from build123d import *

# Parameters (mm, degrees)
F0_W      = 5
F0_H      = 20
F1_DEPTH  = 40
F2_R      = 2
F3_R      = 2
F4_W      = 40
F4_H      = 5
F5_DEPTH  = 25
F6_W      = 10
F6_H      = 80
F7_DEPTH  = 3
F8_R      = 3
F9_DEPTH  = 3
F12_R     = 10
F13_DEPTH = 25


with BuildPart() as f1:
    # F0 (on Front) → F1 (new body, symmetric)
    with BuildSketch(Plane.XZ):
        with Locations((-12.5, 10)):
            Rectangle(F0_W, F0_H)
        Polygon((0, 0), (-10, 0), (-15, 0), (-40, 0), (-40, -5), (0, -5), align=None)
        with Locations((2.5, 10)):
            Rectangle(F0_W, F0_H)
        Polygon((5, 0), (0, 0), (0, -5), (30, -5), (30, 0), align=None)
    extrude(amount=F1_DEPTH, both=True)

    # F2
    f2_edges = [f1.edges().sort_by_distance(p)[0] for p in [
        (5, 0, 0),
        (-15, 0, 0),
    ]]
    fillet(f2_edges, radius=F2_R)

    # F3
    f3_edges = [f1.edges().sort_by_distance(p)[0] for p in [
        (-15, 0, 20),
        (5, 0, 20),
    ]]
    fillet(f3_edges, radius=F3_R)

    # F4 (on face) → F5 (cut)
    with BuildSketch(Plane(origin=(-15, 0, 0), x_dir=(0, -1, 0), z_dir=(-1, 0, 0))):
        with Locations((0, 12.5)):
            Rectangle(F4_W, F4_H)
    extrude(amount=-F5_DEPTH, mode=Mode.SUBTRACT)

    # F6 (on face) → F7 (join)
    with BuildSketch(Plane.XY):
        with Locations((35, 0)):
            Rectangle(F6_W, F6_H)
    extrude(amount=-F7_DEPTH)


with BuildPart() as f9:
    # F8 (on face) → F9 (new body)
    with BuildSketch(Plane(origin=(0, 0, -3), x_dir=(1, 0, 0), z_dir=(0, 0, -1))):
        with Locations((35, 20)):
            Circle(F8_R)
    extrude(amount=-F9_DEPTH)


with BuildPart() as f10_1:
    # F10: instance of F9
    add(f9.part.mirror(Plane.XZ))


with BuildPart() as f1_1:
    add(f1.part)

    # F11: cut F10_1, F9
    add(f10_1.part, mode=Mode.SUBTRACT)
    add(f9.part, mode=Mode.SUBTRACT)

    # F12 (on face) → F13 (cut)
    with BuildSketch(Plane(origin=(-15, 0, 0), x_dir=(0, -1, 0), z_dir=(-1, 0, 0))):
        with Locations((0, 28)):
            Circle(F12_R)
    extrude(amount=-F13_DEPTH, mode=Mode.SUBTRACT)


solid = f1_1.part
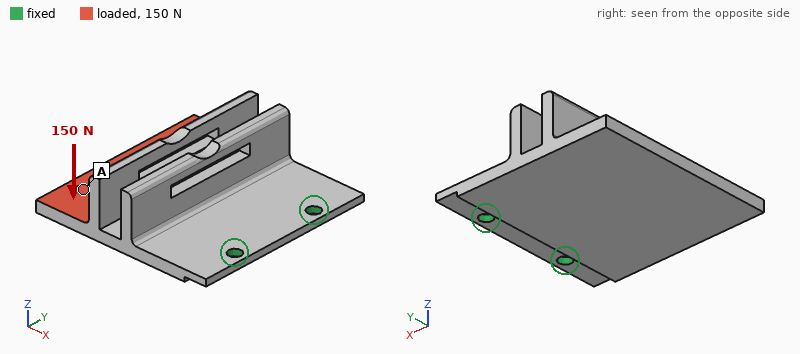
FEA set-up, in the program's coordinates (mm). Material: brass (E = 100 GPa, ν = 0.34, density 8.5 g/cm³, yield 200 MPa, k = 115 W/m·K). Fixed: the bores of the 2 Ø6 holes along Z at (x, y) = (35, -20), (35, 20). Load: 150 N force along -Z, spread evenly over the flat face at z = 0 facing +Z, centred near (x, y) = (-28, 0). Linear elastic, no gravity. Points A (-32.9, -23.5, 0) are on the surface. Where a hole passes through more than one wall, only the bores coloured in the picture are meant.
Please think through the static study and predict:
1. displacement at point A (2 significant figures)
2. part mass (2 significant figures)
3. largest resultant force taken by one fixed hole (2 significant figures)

0.34 mm
370 g
76 N
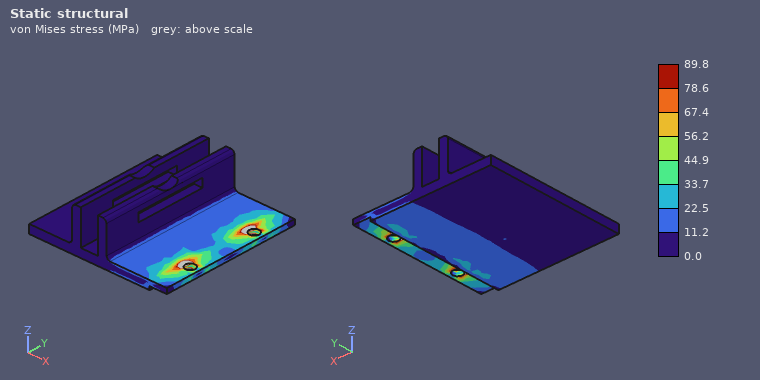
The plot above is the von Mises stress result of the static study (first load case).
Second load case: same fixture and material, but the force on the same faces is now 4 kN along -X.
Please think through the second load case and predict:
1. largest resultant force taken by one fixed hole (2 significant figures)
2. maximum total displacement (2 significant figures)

2.0 kN
0.40 mm
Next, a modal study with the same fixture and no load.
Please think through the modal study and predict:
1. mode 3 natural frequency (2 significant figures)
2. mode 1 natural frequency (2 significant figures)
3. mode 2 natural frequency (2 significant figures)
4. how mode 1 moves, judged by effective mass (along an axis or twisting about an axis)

2000 Hz
280 Hz
800 Hz
along Z
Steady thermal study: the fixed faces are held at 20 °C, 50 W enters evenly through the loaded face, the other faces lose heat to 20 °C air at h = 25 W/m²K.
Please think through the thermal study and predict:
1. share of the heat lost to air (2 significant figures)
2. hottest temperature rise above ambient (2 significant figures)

33 %
61 K
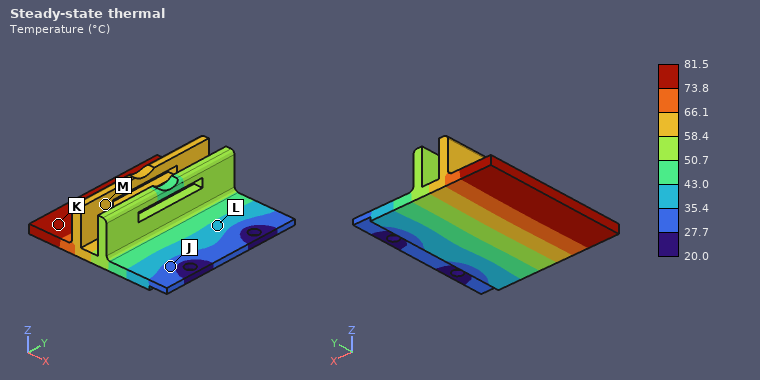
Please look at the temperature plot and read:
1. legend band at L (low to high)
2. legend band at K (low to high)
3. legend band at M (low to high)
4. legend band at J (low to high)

35.4 to 43.0 °C
73.8 to 81.5 °C
58.4 to 66.1 °C
27.7 to 35.4 °C
